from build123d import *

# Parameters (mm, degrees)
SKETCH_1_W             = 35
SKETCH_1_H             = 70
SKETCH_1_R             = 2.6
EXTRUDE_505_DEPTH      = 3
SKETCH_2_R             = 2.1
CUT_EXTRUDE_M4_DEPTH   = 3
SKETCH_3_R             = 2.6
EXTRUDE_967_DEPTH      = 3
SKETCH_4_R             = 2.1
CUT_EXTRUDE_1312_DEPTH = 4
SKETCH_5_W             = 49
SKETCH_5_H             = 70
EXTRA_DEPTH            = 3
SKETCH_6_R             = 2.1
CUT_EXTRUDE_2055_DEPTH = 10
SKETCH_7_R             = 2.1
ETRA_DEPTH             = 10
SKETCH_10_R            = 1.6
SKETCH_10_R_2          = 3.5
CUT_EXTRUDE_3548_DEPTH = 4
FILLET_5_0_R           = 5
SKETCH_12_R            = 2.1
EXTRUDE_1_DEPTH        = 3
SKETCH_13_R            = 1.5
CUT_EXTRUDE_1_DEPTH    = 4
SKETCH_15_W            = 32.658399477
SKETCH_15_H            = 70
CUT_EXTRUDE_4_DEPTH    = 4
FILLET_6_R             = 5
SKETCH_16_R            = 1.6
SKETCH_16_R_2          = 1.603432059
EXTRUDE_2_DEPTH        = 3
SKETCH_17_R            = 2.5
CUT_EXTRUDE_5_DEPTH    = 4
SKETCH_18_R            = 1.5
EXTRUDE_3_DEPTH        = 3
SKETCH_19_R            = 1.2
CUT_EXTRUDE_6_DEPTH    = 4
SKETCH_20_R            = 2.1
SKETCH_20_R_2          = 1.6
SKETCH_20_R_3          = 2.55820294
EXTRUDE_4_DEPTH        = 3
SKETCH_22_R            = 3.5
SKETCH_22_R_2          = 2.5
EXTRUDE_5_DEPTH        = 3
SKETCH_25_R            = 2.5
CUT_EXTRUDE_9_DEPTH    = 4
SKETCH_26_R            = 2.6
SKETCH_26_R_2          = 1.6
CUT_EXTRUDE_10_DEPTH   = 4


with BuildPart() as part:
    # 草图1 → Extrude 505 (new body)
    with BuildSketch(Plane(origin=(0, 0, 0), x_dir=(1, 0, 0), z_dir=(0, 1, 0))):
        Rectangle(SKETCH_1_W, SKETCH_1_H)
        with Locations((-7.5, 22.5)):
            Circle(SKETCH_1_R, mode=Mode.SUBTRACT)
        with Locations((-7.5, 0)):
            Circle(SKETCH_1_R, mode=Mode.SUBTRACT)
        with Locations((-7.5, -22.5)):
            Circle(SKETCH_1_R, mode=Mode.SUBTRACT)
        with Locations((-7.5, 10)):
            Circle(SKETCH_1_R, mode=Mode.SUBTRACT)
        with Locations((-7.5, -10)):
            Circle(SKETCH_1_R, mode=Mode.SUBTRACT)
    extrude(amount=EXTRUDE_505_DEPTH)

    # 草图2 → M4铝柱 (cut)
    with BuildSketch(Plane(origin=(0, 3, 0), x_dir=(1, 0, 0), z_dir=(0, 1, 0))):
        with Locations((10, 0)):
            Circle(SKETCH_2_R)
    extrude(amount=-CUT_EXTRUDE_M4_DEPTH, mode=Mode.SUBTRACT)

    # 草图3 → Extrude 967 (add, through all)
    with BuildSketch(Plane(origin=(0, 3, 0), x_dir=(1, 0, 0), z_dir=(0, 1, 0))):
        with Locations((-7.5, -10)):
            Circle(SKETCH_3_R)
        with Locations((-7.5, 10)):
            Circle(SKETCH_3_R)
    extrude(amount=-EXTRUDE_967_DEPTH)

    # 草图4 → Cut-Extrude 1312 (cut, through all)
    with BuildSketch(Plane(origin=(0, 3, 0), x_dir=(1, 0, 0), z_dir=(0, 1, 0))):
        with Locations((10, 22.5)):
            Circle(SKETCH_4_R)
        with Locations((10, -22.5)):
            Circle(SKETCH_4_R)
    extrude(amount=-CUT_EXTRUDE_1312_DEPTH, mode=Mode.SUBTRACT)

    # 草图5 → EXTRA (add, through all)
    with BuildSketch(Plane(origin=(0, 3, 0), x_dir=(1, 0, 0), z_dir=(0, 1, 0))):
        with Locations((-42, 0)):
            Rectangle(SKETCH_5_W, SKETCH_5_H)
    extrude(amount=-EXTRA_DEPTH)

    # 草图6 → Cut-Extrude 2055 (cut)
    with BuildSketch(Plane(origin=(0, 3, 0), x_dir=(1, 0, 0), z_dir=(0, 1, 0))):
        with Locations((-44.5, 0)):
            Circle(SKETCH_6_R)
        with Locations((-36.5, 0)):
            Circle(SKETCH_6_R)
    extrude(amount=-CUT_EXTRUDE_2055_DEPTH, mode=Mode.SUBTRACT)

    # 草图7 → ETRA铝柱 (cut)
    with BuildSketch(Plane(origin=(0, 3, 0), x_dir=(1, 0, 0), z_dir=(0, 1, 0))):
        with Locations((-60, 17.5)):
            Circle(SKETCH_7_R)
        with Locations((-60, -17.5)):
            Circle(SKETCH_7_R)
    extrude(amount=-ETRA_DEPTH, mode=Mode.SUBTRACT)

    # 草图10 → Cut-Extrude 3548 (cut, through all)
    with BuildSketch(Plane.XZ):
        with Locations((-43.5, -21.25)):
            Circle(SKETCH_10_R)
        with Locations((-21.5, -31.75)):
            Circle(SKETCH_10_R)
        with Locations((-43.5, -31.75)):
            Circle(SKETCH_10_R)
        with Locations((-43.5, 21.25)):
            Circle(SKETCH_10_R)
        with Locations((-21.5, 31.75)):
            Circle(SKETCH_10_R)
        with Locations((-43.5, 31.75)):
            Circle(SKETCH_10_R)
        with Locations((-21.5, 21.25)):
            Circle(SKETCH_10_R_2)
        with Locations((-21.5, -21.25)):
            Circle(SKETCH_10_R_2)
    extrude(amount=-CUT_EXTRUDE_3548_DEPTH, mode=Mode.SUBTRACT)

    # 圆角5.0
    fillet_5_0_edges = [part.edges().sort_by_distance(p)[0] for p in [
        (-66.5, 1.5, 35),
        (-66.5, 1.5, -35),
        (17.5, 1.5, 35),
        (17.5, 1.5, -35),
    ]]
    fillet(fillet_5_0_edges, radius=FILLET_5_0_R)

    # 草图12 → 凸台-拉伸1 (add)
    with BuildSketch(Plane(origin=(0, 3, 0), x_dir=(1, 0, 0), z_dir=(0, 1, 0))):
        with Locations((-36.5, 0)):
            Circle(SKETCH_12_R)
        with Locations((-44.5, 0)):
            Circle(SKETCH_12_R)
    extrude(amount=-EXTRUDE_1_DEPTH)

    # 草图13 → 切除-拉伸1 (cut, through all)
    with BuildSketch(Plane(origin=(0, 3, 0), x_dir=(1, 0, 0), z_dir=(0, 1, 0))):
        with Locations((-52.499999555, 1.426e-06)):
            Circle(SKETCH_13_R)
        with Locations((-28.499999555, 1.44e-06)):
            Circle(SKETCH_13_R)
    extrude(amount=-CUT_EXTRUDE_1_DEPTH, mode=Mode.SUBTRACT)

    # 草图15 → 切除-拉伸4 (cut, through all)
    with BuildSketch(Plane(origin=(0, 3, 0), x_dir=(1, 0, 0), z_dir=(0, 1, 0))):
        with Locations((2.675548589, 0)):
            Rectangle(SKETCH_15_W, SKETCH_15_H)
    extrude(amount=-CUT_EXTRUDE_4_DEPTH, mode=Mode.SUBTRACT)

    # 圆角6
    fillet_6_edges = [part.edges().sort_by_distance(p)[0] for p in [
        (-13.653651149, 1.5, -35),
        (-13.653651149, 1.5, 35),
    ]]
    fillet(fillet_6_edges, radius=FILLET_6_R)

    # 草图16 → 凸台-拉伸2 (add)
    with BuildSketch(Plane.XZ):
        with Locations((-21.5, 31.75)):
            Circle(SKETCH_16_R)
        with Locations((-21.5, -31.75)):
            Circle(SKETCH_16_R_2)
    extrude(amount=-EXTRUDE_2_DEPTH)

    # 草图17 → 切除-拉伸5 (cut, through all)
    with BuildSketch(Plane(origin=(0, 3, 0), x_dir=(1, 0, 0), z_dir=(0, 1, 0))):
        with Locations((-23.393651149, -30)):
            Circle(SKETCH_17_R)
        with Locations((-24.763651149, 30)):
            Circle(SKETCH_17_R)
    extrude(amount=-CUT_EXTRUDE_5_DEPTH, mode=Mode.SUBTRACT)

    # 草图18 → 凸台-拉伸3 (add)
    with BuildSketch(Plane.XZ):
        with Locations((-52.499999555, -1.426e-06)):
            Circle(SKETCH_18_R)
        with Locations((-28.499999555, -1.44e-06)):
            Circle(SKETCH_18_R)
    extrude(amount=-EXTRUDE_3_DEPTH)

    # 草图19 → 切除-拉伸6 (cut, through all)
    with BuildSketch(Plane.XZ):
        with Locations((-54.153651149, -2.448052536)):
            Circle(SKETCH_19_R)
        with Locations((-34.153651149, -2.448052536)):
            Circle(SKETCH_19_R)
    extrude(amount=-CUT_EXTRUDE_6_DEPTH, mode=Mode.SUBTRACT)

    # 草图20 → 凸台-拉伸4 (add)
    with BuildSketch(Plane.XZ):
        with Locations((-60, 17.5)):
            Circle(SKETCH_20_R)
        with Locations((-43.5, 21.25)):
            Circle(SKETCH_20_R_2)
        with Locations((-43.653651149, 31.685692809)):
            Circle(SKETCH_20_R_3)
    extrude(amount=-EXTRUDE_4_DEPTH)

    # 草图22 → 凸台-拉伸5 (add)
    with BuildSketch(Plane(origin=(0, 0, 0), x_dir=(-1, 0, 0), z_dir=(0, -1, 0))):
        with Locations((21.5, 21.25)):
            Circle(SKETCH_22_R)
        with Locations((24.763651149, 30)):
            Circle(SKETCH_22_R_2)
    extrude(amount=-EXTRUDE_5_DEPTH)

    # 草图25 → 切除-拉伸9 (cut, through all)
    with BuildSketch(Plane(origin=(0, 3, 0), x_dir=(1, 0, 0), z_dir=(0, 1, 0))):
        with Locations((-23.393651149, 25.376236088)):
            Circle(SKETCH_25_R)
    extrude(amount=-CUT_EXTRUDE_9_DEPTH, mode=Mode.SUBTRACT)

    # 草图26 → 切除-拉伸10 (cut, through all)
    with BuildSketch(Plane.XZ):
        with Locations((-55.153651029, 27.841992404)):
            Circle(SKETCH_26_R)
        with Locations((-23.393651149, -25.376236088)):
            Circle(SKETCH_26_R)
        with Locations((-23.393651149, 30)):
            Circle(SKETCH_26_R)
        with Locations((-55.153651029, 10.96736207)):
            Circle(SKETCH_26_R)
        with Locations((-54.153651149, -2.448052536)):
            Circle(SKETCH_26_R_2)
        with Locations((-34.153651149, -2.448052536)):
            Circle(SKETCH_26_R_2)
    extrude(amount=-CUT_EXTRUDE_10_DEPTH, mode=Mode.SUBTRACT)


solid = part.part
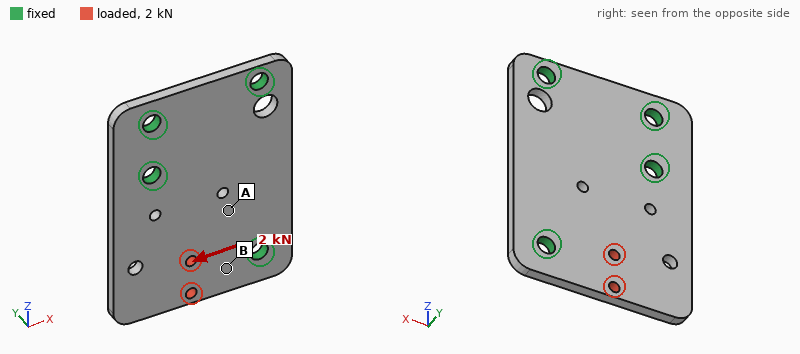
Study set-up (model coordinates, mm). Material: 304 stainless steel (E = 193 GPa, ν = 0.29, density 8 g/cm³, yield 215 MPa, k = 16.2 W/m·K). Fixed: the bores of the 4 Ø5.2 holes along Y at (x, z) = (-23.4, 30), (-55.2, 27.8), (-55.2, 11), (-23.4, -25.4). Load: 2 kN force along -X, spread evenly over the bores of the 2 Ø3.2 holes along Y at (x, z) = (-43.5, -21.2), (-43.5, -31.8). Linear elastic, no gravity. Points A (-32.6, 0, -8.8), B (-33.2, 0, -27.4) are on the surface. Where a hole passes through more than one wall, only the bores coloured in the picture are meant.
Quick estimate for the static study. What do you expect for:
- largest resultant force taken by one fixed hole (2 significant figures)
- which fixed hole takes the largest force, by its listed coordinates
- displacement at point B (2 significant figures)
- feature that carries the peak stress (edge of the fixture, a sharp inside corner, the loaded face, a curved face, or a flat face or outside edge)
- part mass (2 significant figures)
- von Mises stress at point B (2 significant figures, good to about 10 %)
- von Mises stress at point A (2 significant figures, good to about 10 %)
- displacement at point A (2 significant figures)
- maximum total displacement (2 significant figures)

1.7 kN
(-23.4, -25.4)
1.8 µm
the loaded face
84 g
38 MPa
6.3 MPa
1.4 µm
4.7 µm
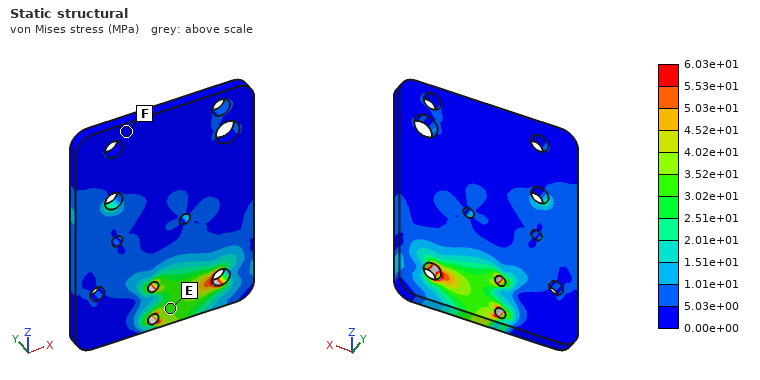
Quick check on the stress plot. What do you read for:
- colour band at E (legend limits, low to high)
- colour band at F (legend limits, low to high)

3.02e+01 to 3.52e+01 MPa
0.00e+00 to 5.03e+00 MPa
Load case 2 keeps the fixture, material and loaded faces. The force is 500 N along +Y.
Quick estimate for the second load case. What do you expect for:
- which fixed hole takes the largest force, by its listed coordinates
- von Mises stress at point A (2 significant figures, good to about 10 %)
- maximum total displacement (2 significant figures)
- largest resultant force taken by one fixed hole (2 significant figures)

(-23.4, -25.4)
38 MPa
0.13 mm
410 N
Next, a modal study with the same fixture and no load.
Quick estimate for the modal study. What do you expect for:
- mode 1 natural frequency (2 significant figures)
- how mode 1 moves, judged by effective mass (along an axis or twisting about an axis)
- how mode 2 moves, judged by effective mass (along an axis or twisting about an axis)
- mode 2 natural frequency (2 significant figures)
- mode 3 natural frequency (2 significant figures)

2500 Hz
along Y
along Y
5500 Hz
7900 Hz
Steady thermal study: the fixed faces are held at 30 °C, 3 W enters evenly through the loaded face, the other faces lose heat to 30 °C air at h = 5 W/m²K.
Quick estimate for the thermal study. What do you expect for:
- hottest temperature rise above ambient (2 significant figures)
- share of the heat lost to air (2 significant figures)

41 K
12 %
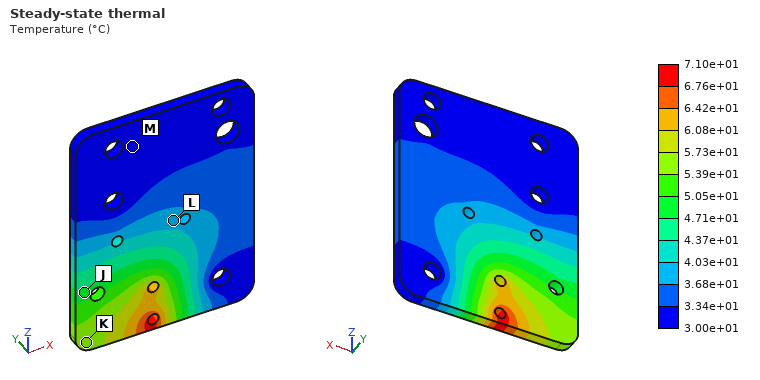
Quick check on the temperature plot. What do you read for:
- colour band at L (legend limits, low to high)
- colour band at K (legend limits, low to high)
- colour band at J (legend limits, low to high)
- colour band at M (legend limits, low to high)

3.68e+01 to 4.03e+01 °C
5.39e+01 to 5.73e+01 °C
4.71e+01 to 5.05e+01 °C
3.00e+01 to 3.34e+01 °C
